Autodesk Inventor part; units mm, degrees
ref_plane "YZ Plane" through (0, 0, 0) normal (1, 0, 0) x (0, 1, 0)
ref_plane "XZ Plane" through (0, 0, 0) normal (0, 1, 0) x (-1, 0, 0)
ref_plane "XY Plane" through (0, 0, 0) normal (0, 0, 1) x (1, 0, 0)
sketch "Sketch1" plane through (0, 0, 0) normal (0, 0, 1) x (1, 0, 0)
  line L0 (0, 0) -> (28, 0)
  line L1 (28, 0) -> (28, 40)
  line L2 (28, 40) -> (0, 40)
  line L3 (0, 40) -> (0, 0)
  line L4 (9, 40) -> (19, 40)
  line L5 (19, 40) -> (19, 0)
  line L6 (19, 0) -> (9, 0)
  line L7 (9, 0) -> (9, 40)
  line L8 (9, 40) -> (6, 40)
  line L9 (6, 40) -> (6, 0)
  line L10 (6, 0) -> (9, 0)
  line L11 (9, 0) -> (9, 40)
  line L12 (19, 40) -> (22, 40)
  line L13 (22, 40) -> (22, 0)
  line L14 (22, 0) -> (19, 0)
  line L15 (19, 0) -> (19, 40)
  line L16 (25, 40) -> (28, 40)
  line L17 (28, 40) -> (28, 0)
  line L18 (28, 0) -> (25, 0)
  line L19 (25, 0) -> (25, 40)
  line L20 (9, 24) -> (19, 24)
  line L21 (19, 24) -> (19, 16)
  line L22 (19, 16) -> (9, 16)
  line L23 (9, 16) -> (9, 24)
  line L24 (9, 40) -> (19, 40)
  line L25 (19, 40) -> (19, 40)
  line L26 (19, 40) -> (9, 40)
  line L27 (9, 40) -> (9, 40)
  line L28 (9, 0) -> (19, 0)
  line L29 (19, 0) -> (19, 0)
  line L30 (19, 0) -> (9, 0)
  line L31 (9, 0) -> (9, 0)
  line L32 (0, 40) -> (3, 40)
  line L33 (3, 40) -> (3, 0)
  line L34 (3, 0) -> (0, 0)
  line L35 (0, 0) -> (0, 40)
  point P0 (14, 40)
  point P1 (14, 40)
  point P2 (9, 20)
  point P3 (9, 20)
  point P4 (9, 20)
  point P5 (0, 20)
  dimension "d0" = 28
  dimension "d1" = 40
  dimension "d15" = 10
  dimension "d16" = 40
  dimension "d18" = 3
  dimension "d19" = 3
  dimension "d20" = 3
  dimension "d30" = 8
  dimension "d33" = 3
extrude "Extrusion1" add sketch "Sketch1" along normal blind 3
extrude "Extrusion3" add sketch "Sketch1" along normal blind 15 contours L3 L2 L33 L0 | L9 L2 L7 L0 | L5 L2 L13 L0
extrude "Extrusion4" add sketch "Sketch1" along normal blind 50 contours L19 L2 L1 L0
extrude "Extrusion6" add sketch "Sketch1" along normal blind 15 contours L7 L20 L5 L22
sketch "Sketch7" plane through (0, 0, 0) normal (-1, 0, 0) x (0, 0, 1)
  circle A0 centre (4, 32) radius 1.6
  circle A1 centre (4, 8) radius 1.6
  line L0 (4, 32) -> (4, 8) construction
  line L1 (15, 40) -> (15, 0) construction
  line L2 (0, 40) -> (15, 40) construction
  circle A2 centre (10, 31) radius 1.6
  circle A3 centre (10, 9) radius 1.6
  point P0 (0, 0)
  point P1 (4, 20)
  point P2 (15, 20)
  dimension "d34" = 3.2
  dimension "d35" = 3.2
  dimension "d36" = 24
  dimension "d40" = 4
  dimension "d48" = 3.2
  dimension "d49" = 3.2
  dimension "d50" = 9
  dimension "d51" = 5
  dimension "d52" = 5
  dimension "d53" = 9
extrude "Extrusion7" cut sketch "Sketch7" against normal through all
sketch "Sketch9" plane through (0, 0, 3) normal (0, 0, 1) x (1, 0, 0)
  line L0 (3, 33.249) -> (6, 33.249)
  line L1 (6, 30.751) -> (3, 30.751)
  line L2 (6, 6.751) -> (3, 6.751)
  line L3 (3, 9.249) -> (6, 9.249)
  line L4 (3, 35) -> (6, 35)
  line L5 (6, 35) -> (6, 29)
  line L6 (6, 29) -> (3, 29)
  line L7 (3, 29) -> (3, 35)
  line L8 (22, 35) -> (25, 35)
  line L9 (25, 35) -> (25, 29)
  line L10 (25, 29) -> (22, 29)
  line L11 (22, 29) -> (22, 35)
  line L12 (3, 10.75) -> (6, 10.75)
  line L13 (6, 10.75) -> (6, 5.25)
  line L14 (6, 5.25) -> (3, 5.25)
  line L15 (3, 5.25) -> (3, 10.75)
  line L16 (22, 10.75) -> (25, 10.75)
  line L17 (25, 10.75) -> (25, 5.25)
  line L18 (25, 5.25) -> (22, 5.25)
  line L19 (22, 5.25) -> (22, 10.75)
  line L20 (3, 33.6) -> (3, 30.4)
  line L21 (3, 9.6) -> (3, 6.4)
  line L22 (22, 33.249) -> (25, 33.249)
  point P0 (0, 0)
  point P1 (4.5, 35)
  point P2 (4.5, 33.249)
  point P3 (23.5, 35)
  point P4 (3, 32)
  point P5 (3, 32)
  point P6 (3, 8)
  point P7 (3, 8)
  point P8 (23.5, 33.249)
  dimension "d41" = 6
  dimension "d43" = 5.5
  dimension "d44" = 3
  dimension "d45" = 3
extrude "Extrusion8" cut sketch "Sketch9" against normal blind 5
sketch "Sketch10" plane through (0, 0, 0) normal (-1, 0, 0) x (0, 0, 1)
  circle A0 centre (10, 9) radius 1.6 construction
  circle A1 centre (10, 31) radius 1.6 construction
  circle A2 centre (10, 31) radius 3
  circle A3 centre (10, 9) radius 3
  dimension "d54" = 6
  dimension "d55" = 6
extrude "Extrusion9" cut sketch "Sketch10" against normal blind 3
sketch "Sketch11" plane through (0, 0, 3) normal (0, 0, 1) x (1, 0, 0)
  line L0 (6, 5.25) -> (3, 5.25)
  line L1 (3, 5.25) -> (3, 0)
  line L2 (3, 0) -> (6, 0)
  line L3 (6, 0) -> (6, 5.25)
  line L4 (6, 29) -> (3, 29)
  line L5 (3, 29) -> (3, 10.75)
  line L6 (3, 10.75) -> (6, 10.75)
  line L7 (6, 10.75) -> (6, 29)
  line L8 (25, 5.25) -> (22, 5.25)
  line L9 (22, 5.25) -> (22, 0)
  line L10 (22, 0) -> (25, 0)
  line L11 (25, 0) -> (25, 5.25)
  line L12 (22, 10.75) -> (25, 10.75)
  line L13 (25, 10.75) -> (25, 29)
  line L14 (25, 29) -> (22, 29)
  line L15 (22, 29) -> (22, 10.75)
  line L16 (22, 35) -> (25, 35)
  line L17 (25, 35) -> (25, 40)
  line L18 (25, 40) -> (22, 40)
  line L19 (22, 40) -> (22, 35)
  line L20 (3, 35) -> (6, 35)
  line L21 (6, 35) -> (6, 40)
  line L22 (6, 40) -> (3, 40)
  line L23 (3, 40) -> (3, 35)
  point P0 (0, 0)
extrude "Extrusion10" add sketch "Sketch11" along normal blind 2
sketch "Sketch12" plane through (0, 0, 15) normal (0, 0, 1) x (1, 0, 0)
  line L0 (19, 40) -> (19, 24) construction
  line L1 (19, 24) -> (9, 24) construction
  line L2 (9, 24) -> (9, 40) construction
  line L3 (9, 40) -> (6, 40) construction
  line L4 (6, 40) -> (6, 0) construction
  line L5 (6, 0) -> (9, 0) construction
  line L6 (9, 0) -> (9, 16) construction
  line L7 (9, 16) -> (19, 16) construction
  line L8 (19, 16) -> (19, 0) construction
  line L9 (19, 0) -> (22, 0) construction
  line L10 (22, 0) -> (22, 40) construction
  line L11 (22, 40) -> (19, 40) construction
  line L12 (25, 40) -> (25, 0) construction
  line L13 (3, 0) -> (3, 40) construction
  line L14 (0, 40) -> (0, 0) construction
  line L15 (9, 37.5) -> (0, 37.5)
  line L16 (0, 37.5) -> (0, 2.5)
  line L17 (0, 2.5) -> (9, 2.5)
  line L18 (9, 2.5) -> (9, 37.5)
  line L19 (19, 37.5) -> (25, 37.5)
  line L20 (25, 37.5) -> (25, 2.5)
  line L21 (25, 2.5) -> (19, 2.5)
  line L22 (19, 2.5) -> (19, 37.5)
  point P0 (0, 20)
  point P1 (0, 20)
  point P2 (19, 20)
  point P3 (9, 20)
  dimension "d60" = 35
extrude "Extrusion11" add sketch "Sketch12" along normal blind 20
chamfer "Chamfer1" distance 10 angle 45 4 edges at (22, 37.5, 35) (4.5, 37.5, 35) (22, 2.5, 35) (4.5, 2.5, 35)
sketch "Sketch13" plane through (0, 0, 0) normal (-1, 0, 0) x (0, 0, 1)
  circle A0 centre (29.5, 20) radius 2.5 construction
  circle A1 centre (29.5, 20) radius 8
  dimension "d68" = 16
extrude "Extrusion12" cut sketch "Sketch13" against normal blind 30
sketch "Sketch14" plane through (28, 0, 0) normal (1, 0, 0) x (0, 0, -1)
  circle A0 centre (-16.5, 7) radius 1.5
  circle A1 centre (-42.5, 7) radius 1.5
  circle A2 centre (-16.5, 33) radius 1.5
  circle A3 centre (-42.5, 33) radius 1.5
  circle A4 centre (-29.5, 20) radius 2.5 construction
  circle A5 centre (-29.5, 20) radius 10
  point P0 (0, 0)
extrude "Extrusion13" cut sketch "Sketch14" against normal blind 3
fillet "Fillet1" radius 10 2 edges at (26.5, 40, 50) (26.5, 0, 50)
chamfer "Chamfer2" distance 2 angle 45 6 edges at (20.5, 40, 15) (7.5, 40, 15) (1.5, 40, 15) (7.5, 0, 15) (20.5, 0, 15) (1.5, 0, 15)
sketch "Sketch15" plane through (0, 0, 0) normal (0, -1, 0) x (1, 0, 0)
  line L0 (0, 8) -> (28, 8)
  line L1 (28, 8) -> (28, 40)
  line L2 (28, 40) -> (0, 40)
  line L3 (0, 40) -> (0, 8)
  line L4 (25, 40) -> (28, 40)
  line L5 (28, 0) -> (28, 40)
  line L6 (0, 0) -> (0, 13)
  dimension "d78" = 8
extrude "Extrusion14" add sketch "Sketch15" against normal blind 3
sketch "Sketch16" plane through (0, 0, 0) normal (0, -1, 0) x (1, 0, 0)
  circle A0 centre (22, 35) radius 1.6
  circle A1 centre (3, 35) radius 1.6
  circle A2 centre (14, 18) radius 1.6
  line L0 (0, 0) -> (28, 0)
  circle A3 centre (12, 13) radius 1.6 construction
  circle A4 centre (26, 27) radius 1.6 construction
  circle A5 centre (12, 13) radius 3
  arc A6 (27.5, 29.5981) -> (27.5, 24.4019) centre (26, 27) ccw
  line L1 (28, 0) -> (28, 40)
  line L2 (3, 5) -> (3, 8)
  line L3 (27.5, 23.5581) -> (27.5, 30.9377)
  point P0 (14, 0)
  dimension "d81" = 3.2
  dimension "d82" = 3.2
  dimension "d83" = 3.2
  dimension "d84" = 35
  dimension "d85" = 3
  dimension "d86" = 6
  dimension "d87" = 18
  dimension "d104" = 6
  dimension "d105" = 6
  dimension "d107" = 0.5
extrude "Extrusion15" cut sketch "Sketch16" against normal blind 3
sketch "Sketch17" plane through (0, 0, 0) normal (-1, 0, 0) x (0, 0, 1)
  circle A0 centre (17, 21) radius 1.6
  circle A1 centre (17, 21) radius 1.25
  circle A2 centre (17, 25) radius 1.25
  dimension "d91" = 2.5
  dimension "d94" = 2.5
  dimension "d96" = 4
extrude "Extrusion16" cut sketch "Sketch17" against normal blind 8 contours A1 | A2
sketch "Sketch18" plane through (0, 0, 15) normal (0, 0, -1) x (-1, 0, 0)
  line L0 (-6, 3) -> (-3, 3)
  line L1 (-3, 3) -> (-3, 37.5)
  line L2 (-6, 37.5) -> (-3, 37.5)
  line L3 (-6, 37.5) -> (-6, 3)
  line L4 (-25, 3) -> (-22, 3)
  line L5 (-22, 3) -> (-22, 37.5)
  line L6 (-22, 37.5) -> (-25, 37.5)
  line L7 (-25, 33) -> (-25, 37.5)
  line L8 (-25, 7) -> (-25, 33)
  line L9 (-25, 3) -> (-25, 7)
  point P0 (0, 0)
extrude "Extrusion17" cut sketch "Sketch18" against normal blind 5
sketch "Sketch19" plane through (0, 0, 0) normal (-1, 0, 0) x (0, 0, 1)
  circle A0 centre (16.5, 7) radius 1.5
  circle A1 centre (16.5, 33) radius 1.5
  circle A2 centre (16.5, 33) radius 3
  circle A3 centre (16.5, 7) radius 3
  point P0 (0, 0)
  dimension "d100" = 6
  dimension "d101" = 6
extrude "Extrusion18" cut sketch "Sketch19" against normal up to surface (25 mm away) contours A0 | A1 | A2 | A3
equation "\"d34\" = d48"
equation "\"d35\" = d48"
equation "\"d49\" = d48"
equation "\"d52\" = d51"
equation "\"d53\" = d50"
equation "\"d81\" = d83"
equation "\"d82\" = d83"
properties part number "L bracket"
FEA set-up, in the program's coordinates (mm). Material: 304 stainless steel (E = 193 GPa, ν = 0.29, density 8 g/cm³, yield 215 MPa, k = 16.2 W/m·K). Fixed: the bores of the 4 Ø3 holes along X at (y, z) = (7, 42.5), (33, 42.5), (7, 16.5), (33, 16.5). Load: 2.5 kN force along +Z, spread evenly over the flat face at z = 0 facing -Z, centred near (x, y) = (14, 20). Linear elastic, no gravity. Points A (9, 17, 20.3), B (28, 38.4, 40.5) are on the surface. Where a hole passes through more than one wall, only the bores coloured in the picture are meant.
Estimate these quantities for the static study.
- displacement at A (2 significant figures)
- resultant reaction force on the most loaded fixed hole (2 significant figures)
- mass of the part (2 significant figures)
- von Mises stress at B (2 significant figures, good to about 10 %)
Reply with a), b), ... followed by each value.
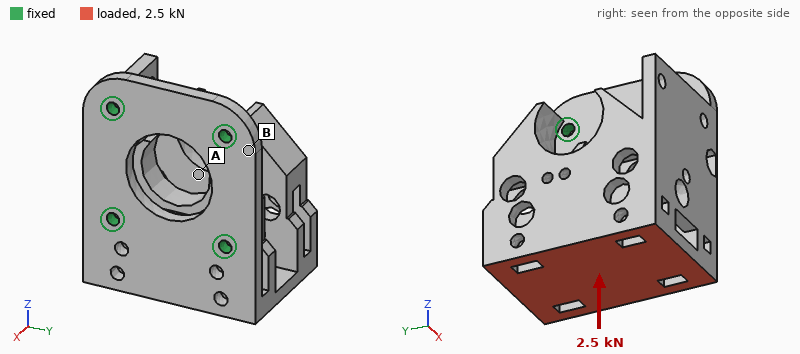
a) 22 µm
b) 1.1 kN
c) 150 g
d) 29 MPa
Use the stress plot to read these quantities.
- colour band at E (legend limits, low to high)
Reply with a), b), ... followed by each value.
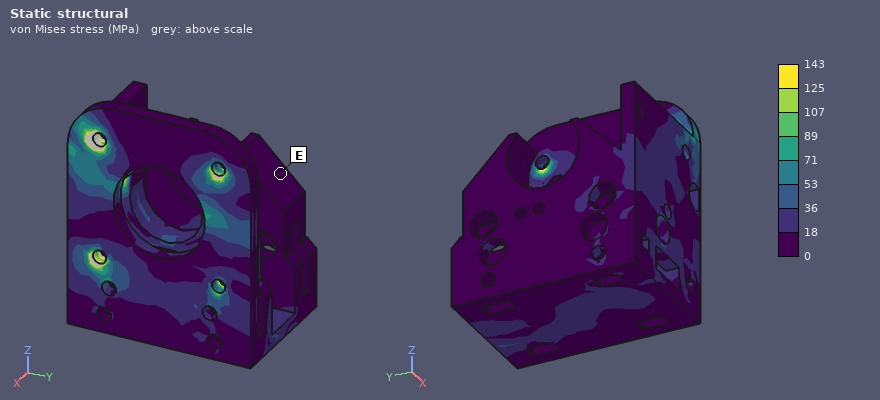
a) 0 to 18 MPa
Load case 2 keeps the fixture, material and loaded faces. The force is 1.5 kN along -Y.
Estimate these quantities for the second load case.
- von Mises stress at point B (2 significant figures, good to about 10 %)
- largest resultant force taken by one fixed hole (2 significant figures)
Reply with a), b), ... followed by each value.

a) 13 MPa
b) 1.2 kN
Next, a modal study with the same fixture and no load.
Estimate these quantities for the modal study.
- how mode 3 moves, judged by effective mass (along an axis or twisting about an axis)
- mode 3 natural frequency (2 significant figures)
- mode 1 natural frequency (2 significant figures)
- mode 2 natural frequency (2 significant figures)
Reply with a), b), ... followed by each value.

a) along X
b) 6400 Hz
c) 3700 Hz
d) 4000 Hz
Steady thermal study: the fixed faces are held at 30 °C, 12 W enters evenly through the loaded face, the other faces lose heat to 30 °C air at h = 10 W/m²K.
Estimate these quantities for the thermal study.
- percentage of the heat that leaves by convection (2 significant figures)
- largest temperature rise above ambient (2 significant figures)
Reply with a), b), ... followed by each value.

a) 34 %
b) 62 K
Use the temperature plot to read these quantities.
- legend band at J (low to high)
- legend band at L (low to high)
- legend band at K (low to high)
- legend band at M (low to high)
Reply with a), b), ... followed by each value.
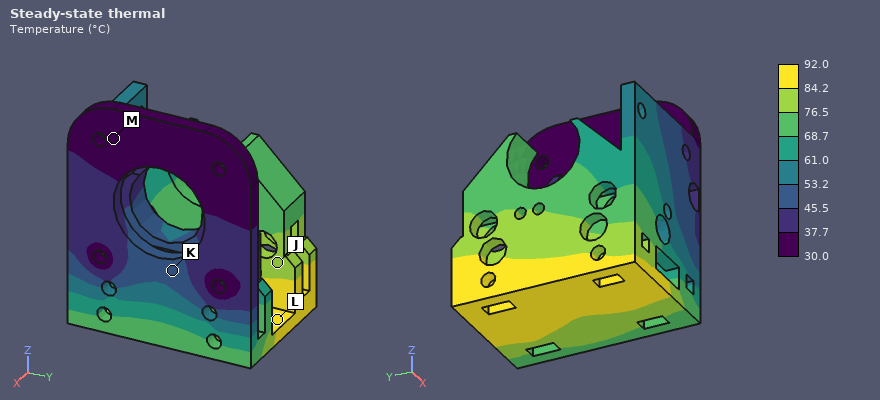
a) 76.5 to 84.2 °C
b) 84.2 to 92.0 °C
c) 45.5 to 53.2 °C
d) 30.0 to 37.7 °C
